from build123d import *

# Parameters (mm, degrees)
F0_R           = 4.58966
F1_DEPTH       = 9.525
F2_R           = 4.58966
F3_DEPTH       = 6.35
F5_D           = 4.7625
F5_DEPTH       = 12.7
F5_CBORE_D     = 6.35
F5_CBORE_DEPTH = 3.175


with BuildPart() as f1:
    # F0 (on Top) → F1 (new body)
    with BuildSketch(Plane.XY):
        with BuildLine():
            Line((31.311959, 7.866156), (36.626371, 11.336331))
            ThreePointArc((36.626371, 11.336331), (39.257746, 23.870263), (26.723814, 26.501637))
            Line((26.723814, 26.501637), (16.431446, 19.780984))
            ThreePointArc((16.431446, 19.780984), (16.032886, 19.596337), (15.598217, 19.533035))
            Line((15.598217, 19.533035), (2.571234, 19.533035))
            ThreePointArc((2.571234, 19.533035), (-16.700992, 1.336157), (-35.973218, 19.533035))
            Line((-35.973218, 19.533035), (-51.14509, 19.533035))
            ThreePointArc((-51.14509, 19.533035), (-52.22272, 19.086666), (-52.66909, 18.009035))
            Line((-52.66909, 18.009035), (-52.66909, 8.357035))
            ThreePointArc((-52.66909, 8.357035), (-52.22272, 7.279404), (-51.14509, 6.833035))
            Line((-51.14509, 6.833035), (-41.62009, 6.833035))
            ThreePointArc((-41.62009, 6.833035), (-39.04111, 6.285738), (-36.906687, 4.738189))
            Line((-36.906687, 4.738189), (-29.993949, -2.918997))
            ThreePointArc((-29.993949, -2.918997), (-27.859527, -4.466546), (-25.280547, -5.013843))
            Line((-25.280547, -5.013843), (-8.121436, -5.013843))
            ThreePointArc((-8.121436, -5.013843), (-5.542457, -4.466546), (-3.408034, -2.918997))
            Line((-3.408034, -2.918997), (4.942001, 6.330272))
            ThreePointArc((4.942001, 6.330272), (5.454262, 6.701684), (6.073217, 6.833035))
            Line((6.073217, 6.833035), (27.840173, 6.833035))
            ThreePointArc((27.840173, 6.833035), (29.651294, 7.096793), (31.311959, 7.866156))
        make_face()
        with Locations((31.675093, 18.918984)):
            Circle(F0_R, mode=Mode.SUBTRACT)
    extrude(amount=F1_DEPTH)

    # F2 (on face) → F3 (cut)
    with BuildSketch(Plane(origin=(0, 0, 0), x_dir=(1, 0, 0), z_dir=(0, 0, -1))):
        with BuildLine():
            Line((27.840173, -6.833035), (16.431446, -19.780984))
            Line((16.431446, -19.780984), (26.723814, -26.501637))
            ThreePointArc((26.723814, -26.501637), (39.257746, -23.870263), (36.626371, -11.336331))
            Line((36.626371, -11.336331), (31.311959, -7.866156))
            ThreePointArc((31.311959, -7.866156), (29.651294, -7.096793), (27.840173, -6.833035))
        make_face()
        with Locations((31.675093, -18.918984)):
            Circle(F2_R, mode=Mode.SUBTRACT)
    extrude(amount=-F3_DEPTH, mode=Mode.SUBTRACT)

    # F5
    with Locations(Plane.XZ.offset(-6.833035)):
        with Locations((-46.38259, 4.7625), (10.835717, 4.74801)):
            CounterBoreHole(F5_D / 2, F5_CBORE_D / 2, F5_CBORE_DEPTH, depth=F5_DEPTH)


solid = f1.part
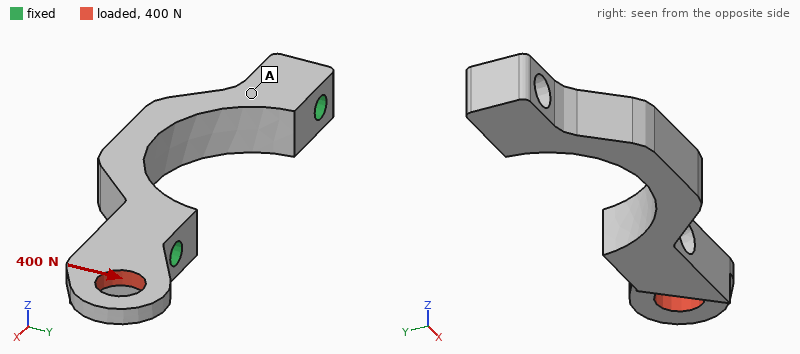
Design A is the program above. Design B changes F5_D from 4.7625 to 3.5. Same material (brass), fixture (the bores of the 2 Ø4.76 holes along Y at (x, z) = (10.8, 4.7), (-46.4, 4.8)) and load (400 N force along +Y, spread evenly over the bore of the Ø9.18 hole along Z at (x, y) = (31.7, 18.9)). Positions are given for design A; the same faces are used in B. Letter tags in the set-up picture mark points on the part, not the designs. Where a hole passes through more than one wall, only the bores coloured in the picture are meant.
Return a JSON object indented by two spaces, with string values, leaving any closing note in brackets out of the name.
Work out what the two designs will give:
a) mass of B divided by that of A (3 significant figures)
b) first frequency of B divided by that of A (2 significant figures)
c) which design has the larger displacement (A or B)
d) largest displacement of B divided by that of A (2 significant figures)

{
  "mass of B divided by that of A": "1.02",
  "first frequency of B divided by that of A": "0.97",
  "which design has the larger displacement": "B",
  "largest displacement of B divided by that of A": "1.1"
}
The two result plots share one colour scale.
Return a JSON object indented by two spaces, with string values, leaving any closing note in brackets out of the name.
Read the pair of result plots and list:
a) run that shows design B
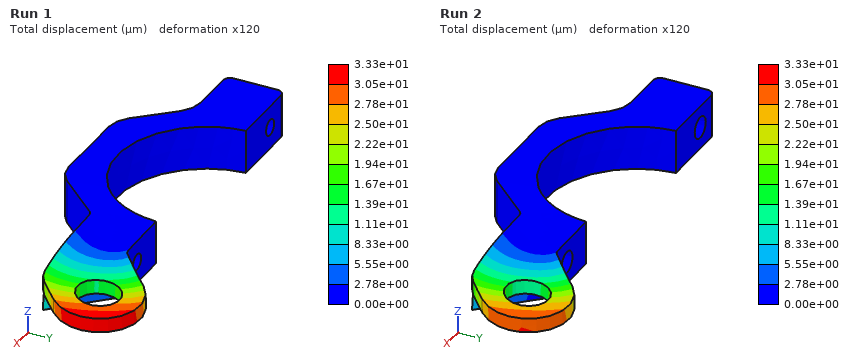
{
  "run that shows design B": "Run 1"
}
